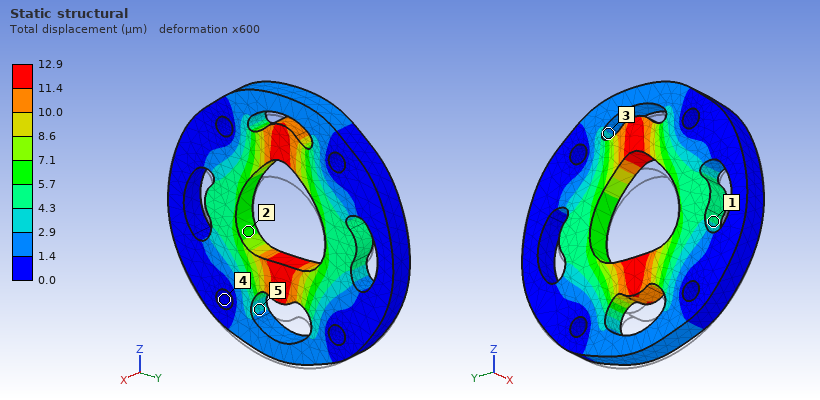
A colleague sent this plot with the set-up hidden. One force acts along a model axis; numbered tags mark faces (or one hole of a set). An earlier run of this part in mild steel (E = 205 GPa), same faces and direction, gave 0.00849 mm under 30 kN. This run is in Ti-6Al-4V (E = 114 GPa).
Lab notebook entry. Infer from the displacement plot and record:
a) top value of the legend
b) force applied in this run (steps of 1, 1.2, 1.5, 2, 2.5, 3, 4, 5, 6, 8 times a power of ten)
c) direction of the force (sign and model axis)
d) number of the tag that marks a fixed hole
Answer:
12.9 µm
25 kN
+Z
4
